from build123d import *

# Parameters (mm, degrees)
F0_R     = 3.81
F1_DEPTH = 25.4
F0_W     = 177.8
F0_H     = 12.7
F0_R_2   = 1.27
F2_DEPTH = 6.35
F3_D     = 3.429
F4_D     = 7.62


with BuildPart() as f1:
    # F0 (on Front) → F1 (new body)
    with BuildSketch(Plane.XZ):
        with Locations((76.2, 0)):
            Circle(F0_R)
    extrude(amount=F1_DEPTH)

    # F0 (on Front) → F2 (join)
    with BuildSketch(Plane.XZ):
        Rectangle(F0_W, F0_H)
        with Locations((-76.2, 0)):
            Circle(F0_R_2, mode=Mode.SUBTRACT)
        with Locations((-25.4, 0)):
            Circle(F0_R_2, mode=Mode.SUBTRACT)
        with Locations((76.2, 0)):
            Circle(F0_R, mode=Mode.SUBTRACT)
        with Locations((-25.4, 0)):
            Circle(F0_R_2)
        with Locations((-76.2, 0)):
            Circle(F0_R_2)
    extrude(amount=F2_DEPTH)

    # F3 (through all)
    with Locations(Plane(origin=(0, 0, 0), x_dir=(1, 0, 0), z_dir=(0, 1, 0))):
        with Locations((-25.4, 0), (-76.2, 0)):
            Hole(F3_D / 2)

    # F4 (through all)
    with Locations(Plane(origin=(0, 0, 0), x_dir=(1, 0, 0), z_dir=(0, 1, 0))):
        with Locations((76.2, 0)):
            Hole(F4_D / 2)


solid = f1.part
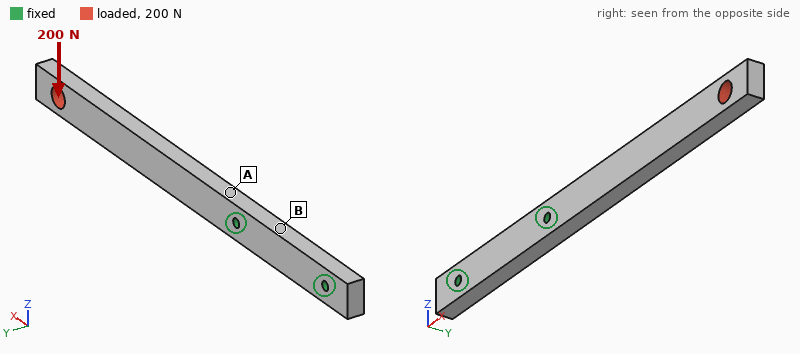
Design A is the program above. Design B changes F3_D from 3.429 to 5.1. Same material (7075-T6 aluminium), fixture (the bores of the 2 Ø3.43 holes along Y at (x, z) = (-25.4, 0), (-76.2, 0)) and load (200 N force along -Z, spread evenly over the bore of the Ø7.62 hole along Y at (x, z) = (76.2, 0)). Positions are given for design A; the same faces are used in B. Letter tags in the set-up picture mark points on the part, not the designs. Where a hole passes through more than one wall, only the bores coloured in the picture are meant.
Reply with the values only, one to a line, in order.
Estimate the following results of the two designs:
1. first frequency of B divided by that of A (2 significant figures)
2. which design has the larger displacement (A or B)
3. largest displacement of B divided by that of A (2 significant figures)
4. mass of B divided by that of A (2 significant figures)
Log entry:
1.0
A
0.91
0.99
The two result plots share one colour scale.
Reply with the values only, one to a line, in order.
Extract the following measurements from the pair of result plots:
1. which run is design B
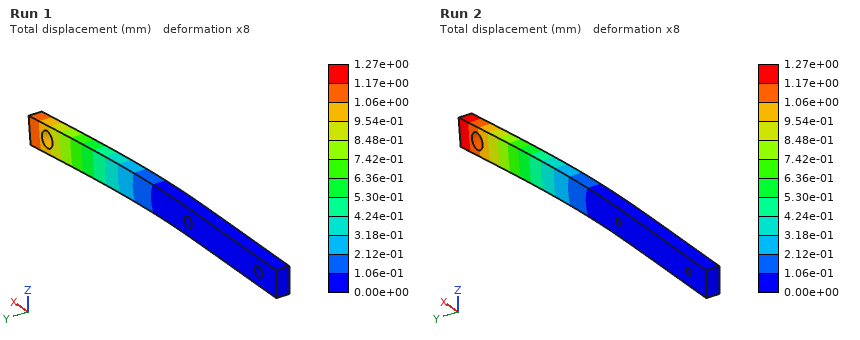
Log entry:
Run 1
